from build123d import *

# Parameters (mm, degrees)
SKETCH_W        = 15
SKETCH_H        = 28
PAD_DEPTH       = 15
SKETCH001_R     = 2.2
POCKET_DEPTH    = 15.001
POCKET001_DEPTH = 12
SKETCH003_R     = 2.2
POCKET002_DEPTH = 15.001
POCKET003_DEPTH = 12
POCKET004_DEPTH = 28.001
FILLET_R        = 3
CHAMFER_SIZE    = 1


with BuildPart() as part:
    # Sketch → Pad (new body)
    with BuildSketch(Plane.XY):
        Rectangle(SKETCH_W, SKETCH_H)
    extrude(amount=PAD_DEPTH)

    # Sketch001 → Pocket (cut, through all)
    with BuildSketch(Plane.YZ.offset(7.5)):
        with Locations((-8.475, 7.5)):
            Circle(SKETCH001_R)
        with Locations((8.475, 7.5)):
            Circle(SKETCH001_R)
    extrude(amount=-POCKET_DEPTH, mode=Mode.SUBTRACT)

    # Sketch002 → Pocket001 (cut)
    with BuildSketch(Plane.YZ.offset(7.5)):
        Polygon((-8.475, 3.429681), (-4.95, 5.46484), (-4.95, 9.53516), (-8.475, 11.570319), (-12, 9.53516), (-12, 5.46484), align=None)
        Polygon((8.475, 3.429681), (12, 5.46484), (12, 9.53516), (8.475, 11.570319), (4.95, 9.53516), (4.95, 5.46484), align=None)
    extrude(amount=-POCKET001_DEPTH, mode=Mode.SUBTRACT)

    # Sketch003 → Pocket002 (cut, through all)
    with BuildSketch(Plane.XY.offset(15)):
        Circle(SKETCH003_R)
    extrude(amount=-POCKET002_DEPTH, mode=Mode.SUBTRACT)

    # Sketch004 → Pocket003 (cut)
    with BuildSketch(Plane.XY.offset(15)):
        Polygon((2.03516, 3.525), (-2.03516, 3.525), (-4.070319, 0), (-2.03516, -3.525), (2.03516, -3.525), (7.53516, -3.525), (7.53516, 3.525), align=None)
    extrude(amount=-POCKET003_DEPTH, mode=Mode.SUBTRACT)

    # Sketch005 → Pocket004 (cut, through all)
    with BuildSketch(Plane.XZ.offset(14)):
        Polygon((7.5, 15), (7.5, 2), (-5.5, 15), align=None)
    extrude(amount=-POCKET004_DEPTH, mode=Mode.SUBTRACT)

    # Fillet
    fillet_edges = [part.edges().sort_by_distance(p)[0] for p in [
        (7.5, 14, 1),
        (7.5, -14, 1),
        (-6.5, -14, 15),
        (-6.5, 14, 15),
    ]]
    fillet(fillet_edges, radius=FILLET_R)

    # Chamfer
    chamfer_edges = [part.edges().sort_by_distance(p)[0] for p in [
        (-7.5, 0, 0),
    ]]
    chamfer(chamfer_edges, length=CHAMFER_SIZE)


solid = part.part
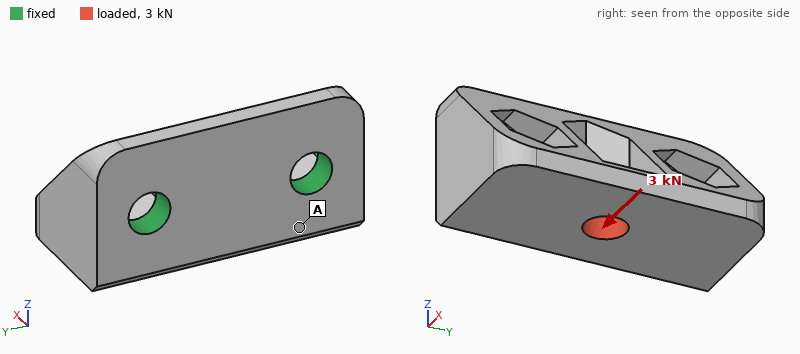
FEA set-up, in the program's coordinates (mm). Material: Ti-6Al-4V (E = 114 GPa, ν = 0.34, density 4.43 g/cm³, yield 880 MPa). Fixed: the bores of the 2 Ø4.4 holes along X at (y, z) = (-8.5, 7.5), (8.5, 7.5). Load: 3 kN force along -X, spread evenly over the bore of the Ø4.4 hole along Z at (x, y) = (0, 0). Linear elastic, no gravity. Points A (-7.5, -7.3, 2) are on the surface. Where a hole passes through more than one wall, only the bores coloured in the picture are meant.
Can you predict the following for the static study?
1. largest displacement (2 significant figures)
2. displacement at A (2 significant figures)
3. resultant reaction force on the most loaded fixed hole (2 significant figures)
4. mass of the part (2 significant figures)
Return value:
42 µm
13 µm
1.6 kN
13 g
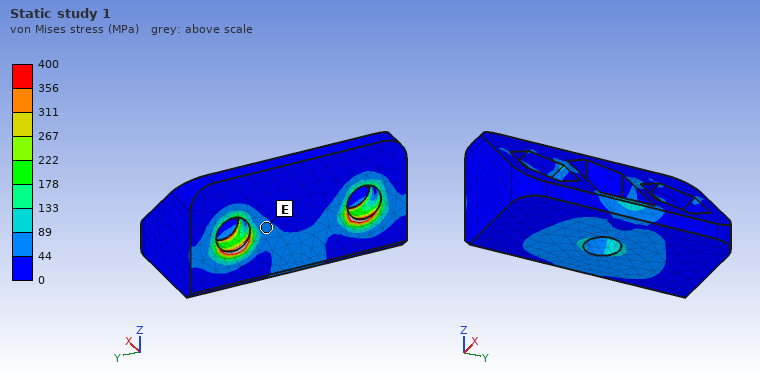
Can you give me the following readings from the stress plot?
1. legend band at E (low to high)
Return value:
44 to 89 MPa
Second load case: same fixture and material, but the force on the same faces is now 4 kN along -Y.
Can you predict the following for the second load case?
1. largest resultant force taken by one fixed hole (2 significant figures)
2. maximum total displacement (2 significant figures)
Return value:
2.6 kN
19 µm
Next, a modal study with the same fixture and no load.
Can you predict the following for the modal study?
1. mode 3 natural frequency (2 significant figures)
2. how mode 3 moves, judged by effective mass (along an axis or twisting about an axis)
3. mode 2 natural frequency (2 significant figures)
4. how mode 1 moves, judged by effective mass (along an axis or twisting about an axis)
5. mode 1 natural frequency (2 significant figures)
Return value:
34 kHz
along Y
23 kHz
along Z
17 kHz
